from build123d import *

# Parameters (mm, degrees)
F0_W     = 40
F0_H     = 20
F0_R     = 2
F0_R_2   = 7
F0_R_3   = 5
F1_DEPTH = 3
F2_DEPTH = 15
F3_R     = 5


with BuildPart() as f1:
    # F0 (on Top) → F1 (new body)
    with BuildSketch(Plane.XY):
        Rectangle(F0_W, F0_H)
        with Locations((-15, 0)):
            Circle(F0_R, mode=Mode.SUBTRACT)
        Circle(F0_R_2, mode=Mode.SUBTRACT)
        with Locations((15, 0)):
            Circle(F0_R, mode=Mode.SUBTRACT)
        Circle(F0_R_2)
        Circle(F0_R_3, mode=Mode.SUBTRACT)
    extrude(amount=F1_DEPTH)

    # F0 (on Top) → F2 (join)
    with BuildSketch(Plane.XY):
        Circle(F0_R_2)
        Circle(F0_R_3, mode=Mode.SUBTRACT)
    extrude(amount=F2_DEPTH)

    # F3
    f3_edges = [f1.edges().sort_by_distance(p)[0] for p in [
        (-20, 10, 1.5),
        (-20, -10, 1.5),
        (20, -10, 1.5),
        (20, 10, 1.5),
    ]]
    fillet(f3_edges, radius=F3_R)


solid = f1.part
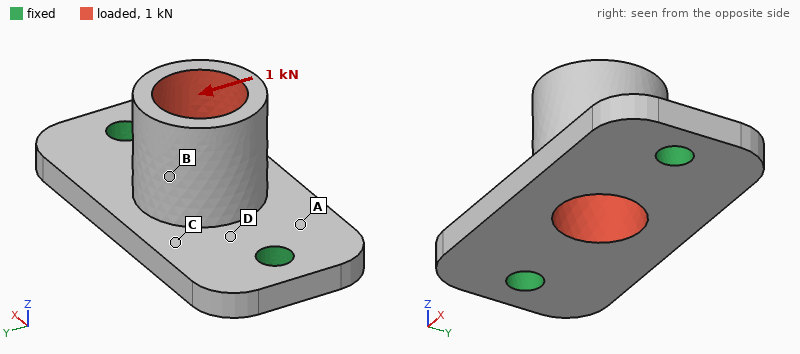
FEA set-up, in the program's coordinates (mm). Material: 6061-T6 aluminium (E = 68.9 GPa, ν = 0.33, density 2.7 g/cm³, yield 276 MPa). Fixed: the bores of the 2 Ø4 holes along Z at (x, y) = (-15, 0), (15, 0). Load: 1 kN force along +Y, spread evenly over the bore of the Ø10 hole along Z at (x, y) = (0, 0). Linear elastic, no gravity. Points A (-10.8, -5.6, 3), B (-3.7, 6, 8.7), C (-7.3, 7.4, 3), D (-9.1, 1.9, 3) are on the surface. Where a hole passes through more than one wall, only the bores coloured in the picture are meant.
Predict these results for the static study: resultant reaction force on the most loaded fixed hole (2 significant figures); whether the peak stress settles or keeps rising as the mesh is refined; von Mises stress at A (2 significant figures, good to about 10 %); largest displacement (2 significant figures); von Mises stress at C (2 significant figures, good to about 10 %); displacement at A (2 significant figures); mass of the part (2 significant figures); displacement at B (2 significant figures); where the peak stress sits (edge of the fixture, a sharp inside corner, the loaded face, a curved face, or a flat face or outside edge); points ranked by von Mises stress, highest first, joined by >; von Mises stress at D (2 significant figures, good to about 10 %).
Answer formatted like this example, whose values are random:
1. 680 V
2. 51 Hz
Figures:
1. 500 N
2. keeps rising
3. 56 MPa
4. 0.10 mm
5. 45 MPa
6. 0.018 mm
7. 7.9 g
8. 0.065 mm
9. edge of the fixture
10. D > A > C > B
11. 90 MPa
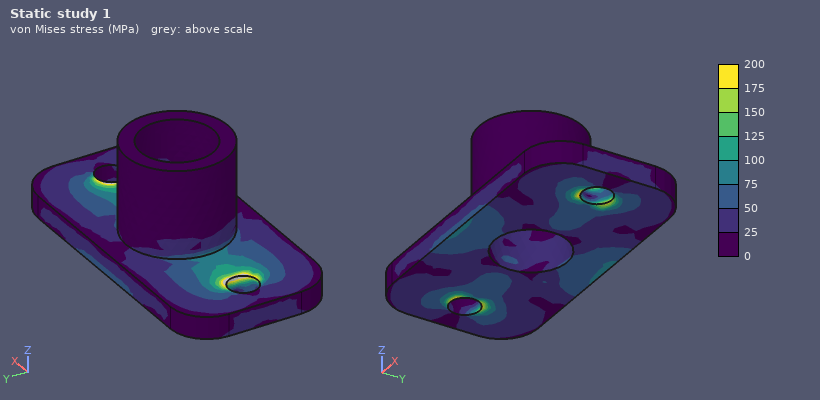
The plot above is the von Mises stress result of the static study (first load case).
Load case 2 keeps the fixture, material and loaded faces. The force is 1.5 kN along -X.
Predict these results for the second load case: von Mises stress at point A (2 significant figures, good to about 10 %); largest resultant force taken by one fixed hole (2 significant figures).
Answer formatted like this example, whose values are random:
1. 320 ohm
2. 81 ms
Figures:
1. 20 MPa
2. 860 N
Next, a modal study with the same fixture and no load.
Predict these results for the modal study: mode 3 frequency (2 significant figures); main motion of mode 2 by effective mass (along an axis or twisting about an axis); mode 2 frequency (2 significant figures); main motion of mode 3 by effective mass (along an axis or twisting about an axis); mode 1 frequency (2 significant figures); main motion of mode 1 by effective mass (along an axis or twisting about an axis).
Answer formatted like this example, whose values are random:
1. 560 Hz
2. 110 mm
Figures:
1. 19 kHz
2. along Z
3. 15 kHz
4. along X
5. 8900 Hz
6. along Y
